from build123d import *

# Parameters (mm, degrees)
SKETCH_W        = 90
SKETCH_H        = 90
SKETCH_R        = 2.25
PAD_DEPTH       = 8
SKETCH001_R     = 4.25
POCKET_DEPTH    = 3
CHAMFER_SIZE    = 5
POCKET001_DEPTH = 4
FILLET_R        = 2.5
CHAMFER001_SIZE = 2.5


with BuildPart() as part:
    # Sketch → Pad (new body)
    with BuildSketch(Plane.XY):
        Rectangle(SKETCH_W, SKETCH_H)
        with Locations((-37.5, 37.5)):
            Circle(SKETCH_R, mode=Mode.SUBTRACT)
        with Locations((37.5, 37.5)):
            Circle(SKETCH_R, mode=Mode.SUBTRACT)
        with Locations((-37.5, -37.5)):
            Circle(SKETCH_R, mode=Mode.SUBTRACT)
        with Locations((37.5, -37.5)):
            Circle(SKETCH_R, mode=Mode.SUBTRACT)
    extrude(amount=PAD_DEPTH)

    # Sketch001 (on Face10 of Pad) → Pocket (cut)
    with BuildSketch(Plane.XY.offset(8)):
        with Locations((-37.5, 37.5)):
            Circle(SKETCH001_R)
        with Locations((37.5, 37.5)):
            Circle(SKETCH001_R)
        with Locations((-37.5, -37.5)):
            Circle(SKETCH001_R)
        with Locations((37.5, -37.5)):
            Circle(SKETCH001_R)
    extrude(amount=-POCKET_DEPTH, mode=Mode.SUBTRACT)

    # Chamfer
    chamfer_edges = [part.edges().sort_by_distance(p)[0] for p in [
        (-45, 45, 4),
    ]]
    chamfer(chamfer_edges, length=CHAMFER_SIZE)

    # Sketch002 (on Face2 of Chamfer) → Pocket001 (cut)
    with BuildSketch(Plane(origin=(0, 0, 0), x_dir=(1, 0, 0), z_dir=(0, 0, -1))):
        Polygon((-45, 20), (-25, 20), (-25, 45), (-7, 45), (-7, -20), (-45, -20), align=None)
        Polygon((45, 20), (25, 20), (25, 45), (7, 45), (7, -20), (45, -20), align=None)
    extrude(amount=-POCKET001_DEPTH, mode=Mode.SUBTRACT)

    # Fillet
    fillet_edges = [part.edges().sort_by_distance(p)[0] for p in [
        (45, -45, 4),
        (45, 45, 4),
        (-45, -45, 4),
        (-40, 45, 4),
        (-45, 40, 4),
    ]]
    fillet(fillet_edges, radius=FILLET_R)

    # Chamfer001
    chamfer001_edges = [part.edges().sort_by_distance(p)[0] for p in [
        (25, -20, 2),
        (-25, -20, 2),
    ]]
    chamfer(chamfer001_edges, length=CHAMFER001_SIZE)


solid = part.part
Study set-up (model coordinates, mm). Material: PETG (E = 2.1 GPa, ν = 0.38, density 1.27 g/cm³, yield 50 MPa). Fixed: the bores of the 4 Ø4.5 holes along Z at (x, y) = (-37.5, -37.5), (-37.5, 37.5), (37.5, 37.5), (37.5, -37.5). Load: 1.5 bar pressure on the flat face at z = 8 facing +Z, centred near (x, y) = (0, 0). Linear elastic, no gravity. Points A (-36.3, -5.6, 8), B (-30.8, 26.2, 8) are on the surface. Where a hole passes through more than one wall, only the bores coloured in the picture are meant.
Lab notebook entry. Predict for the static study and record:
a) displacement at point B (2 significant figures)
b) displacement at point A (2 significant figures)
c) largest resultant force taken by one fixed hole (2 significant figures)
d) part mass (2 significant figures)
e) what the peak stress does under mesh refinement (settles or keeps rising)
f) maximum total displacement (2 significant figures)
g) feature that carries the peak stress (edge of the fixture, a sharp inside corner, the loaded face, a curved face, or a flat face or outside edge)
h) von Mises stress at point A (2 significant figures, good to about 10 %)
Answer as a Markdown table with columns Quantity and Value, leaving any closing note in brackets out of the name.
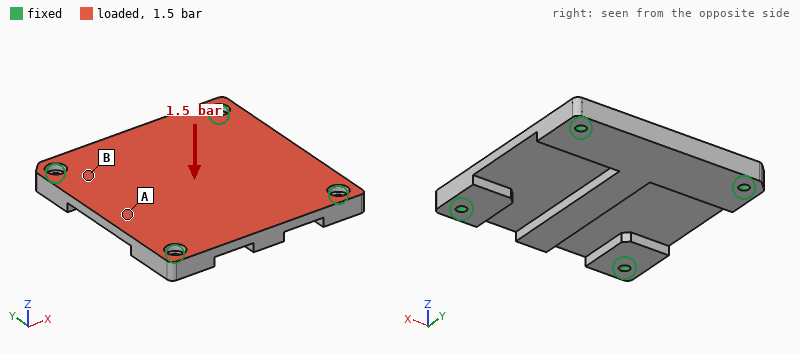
| Quantity | Value |
|---|---|
| displacement at point B | 0.25 mm |
| displacement at point A | 0.49 mm |
| largest resultant force taken by one fixed hole | 570 N |
| part mass | 61 g |
| what the peak stress does under mesh refinement | keeps rising |
| maximum total displacement | 0.85 mm |
| feature that carries the peak stress | edge of the fixture |
| von Mises stress at point A | 8.5 MPa |
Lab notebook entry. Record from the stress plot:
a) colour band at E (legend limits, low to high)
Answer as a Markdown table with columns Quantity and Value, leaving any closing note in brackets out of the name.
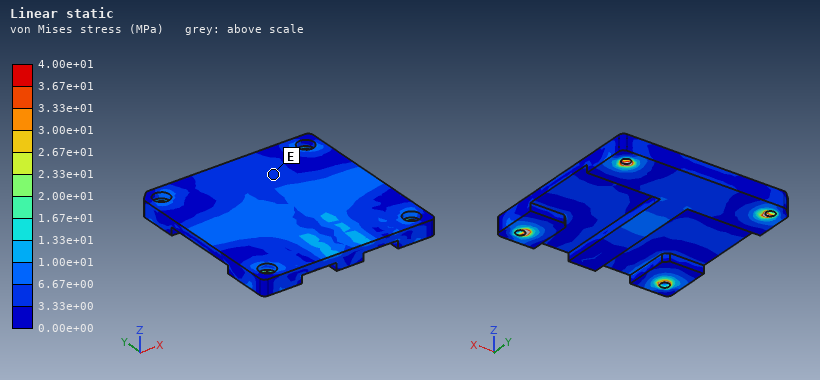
| Quantity | Value |
|---|---|
| colour band at E | 3.33e+00 to 6.67e+00 MPa |
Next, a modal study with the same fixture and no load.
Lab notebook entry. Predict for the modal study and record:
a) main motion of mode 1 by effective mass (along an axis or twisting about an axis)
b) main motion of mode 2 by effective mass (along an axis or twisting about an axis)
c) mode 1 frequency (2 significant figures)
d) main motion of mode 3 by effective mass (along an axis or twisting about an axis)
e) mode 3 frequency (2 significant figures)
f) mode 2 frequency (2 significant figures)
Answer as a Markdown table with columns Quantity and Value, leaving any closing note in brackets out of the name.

| Quantity | Value |
|---|---|
| main motion of mode 1 by effective mass | along Z |
| main motion of mode 2 by effective mass | twisting about X |
| mode 1 frequency | 950 Hz |
| main motion of mode 3 by effective mass | twisting about Y |
| mode 3 frequency | 1700 Hz |
| mode 2 frequency | 1400 Hz |
